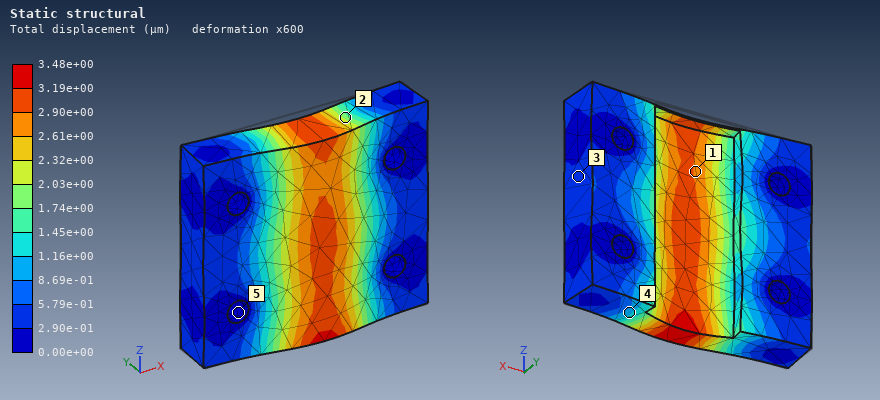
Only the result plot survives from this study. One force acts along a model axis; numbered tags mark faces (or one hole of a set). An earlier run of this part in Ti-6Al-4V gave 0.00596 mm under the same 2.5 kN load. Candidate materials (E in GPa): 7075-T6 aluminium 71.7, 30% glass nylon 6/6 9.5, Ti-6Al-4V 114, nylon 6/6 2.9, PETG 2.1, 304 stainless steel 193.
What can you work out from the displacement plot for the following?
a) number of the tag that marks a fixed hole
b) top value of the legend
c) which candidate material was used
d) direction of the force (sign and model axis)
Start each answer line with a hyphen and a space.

- 5
- 3.48e+00 µm
- 304 stainless steel
- -Y
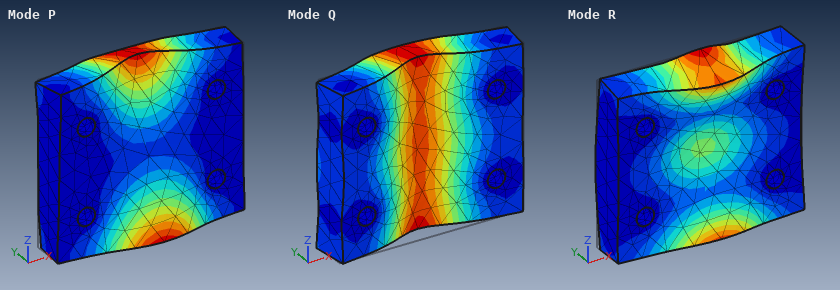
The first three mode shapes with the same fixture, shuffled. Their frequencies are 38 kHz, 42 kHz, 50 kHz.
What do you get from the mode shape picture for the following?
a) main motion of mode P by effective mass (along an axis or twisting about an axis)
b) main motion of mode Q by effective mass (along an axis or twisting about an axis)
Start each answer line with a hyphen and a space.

- twisting about X
- along Y
